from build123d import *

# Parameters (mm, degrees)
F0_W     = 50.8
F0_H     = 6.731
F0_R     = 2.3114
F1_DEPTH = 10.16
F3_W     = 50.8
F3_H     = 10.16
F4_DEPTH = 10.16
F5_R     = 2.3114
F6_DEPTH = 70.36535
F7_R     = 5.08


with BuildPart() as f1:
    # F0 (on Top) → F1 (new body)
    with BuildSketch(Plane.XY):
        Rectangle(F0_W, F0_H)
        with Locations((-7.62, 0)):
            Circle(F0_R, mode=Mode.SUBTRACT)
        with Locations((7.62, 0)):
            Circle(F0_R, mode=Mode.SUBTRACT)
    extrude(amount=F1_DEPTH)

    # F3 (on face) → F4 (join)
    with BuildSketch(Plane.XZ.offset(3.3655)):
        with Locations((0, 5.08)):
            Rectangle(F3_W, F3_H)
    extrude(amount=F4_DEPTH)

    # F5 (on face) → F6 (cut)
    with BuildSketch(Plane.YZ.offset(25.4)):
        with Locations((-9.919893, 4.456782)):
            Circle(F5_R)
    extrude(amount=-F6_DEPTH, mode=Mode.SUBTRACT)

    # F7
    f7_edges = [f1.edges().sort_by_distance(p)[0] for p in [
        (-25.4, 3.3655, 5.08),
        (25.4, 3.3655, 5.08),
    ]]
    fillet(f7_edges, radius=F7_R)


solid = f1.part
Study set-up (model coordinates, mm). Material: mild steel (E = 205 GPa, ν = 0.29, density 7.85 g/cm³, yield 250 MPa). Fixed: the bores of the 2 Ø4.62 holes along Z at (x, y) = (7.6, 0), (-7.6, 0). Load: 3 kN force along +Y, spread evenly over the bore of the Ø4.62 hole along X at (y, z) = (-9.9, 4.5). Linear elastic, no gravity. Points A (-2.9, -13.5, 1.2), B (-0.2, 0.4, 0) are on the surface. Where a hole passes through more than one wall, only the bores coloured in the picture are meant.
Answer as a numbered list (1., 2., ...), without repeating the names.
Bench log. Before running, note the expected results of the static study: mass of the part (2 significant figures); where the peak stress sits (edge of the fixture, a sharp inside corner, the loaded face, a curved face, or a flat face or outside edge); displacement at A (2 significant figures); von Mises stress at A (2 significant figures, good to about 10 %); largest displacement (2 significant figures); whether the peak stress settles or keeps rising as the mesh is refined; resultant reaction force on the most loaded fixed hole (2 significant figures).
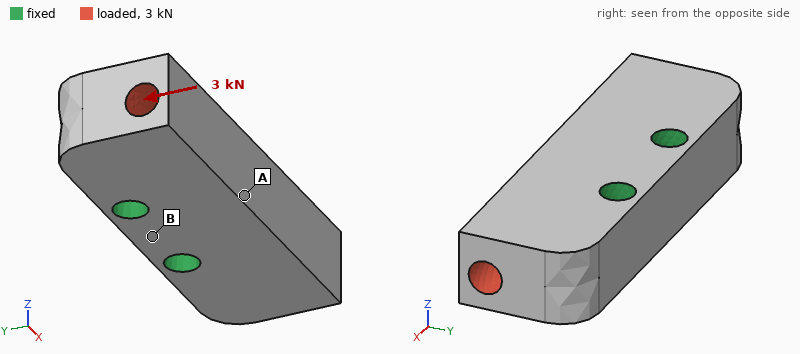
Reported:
1. 58 g
2. edge of the fixture
3. 0.59 µm
4. 15 MPa
5. 3.1 µm
6. keeps rising
7. 1.6 kN
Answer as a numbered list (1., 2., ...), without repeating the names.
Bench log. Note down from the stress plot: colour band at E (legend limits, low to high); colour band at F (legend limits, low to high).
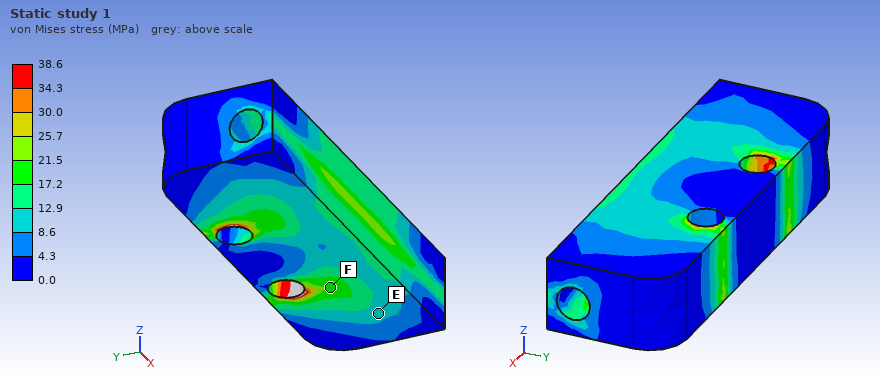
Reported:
1. 8.6 to 12.9 MPa
2. 17.2 to 21.5 MPa
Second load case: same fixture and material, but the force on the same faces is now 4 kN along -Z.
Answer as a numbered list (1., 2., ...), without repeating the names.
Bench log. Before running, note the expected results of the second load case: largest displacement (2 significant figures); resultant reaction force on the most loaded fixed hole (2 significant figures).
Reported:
1. 12 µm
2. 2.0 kN
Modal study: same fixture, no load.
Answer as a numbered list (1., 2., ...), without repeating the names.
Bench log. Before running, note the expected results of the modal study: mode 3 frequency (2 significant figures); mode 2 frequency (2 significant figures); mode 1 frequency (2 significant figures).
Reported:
1. 21 kHz
2. 21 kHz
3. 20 kHz
